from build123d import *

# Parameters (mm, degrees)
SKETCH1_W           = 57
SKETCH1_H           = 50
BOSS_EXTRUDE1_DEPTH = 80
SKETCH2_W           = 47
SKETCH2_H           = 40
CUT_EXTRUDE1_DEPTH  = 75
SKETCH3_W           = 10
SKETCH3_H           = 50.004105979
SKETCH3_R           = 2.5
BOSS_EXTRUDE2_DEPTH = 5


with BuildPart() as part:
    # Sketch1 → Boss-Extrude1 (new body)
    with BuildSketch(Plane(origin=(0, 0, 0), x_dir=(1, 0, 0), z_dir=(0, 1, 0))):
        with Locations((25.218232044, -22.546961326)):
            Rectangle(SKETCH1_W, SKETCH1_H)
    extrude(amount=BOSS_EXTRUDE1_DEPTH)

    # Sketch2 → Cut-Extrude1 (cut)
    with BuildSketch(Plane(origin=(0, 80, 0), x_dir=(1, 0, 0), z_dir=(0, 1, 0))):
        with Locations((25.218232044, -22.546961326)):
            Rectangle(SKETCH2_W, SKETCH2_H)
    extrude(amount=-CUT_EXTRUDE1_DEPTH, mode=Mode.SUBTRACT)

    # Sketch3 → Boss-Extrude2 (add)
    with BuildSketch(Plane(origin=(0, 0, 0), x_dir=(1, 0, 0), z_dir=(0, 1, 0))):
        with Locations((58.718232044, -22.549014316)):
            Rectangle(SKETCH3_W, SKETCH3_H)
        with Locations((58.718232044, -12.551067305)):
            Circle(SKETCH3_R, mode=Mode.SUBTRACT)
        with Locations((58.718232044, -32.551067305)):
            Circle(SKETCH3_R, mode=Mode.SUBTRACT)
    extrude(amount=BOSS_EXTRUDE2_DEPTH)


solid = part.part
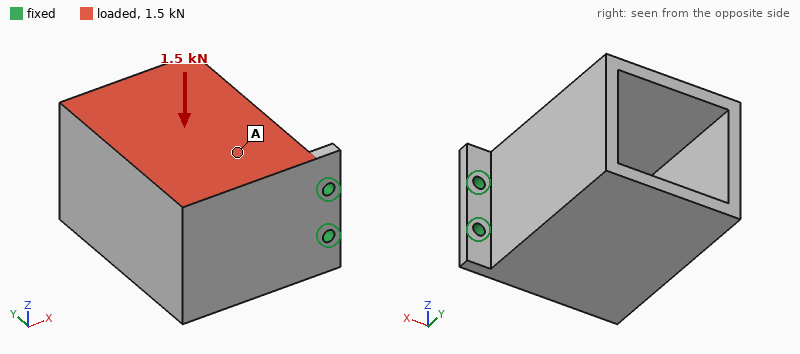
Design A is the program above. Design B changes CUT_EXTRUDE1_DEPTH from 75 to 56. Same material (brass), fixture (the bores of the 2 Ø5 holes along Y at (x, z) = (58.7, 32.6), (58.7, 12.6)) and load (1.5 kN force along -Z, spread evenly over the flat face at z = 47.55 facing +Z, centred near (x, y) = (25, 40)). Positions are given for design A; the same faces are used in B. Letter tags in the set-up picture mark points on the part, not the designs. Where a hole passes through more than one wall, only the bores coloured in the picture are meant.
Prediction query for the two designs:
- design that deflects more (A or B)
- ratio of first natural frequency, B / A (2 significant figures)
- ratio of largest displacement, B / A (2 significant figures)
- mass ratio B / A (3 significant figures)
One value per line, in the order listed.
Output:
A
0.99
0.72
1.40
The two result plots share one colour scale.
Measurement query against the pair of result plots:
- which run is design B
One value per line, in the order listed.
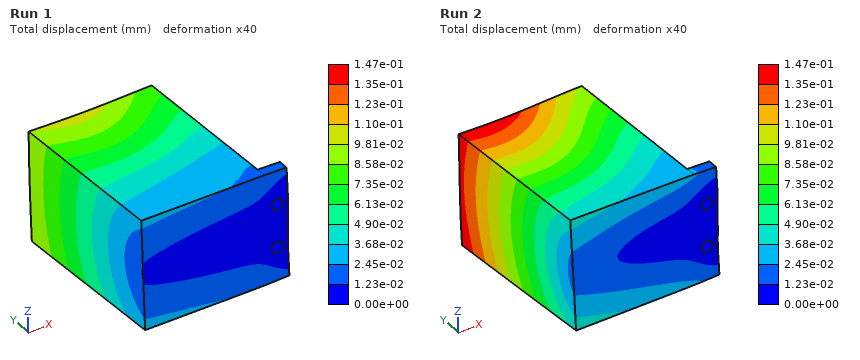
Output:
Run 1
